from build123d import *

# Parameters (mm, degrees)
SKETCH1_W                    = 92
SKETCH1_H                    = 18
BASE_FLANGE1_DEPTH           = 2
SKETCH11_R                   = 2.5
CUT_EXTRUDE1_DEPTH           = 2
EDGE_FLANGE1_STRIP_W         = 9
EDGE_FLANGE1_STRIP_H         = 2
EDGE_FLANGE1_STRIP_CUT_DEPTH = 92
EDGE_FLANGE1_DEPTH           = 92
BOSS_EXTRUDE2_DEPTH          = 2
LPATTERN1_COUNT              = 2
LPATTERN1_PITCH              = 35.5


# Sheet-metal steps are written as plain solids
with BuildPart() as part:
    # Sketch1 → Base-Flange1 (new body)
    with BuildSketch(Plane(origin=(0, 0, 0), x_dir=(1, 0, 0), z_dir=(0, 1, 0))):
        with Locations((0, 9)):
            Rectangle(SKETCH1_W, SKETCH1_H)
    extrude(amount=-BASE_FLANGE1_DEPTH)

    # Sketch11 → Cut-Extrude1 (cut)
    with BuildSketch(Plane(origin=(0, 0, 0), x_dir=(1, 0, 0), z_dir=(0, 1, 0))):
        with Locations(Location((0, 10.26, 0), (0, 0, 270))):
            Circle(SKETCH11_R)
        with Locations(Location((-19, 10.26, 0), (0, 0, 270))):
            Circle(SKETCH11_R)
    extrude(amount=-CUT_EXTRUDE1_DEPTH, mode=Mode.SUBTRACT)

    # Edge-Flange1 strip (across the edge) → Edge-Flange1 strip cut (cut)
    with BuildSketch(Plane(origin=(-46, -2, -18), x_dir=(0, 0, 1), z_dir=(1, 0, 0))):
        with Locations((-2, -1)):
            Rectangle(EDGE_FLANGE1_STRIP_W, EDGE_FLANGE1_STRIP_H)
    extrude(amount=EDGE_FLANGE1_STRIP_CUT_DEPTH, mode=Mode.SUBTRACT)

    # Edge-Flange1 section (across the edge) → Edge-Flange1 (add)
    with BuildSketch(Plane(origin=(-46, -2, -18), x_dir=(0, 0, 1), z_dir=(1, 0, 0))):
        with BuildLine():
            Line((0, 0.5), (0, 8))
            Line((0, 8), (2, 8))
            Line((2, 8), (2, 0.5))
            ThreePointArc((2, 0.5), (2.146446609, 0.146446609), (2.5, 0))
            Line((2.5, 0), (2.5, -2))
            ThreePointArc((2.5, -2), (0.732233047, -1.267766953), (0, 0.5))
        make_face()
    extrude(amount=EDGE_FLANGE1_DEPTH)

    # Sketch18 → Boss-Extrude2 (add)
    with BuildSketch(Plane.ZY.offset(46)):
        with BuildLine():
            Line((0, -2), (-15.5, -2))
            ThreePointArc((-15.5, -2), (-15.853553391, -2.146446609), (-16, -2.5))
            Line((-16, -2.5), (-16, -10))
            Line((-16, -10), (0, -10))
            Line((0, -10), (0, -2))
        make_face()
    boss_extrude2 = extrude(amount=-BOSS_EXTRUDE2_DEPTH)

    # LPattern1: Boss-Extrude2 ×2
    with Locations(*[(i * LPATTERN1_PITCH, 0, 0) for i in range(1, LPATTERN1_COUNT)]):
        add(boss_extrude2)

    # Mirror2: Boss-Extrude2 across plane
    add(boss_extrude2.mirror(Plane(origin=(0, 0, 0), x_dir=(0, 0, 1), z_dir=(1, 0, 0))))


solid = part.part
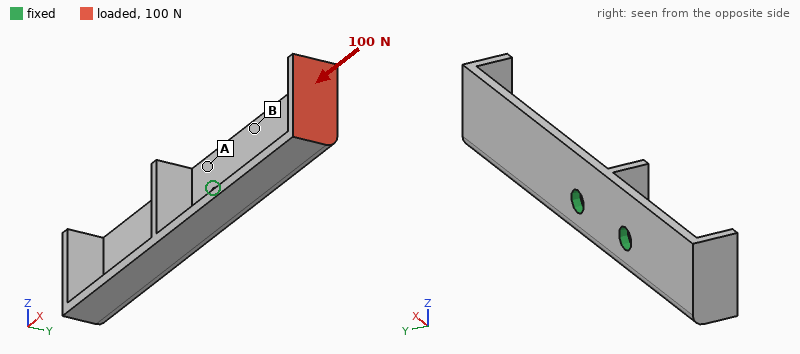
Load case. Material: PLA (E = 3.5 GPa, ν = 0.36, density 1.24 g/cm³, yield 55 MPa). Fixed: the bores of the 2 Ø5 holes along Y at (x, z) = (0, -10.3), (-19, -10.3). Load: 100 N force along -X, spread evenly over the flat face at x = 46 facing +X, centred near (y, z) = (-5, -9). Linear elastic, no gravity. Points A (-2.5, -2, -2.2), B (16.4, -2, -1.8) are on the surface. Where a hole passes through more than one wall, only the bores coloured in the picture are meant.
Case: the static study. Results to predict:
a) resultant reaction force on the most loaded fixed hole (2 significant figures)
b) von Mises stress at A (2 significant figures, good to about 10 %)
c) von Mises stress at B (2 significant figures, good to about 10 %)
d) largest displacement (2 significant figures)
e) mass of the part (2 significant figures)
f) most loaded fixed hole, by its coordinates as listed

62 N
2.7 MPa
6.6 MPa
0.95 mm
6.6 g
(0, -10.3)
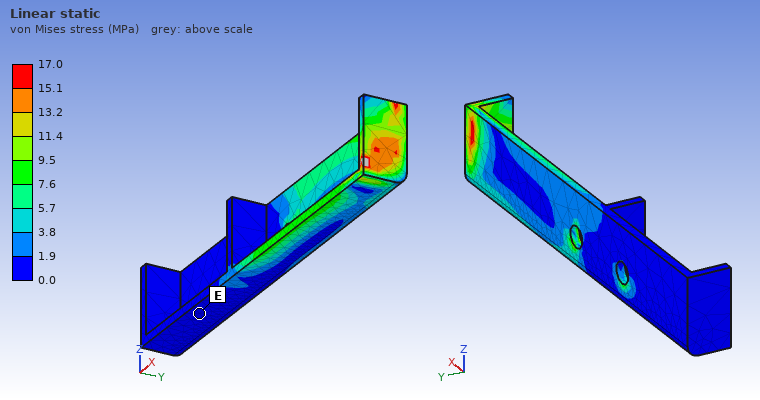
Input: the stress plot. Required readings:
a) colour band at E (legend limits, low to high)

0.0 to 1.9 MPa
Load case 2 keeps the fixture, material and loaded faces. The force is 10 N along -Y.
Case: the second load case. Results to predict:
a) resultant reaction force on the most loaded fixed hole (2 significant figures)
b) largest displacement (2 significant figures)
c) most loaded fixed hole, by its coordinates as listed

37 N
1.0 mm
(0, -10.3)
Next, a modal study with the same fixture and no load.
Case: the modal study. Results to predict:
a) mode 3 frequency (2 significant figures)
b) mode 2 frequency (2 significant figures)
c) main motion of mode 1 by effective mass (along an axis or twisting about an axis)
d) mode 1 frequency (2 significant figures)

1200 Hz
890 Hz
along Y
550 Hz
